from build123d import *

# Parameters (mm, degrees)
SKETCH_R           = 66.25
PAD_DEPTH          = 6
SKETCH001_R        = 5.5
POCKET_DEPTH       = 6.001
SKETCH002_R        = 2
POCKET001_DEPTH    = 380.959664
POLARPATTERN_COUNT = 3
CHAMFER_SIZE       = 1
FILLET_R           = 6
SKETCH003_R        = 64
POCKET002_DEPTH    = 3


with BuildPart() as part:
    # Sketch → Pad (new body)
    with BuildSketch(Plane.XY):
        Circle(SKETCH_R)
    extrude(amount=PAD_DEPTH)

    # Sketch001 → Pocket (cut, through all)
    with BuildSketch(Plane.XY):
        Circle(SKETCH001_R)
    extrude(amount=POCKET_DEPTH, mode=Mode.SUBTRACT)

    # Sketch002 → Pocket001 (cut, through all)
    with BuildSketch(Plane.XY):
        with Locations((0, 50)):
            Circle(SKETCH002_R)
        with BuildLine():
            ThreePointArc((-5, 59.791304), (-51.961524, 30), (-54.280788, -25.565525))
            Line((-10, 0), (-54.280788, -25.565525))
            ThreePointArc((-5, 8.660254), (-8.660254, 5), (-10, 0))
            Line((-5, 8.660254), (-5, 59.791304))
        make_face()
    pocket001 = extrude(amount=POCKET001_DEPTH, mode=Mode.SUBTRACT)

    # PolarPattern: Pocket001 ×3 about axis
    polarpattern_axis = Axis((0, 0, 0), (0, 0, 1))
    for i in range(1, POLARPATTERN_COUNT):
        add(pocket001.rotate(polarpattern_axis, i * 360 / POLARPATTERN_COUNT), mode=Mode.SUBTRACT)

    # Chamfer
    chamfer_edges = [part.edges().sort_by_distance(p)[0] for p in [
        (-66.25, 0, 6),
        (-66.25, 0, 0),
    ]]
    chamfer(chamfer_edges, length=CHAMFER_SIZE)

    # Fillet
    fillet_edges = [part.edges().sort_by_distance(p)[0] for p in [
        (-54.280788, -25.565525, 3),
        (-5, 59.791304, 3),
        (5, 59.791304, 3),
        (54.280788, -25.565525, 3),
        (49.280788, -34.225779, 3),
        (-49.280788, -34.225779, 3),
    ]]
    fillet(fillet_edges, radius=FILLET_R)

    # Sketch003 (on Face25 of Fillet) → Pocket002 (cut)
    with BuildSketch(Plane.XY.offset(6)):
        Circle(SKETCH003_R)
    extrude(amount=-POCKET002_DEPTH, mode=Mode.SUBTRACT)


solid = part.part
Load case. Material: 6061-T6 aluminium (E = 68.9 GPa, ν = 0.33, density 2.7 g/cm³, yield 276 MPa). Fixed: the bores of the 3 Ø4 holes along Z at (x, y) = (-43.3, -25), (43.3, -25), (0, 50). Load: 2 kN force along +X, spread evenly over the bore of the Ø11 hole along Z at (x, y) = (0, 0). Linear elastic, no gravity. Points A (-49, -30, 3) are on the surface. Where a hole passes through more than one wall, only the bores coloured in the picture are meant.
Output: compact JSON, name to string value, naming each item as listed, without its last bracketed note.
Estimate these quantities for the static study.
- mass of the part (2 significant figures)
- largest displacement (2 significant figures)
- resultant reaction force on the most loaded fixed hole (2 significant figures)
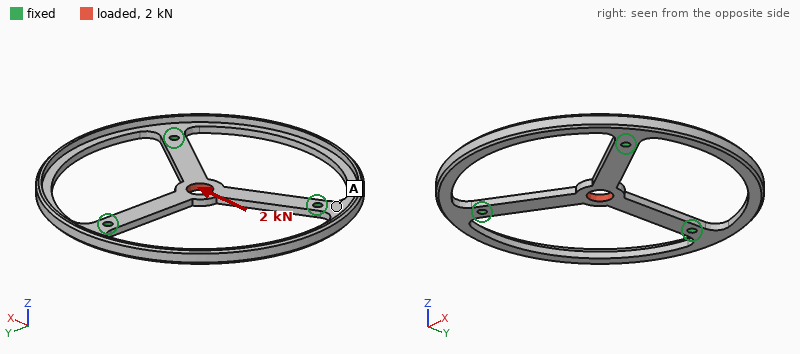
{"mass of the part": "41 g", "largest displacement": "53 µm", "resultant reaction force on the most loaded fixed hole": "1.2 kN"}
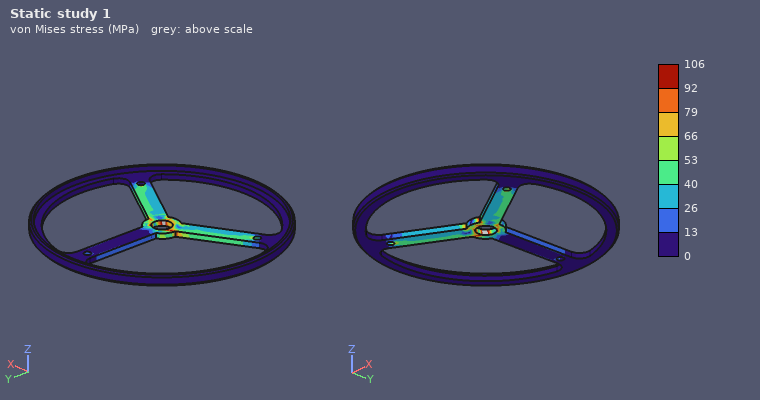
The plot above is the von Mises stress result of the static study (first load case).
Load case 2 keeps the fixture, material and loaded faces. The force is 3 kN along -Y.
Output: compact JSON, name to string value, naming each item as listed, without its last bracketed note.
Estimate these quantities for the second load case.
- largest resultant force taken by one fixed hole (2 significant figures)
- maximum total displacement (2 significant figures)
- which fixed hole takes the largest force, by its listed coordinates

{"largest resultant force taken by one fixed hole": "2.0 kN", "maximum total displacement": "82 µm", "which fixed hole takes the largest force, by its listed coordinates": "(0, 50)"}
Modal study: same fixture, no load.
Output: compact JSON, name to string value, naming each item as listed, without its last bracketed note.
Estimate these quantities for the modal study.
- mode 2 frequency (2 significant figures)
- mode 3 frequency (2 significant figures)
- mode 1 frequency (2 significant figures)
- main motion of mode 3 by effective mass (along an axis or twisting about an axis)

{"mode 2 frequency": "910 Hz", "mode 3 frequency": "1400 Hz", "mode 1 frequency": "910 Hz", "main motion of mode 3 by effective mass": "along Z"}
